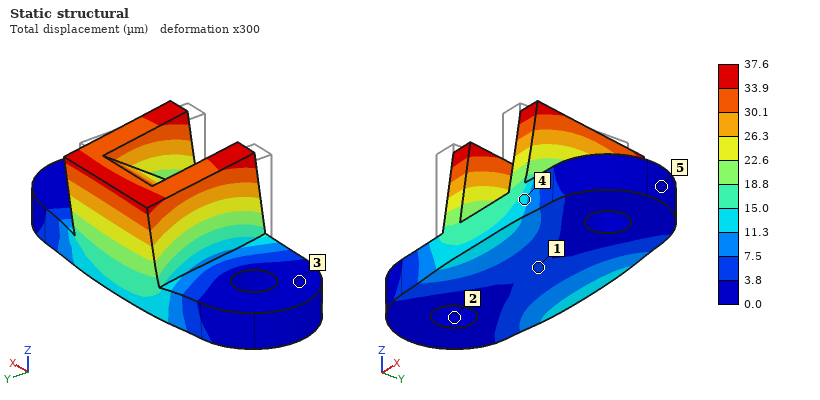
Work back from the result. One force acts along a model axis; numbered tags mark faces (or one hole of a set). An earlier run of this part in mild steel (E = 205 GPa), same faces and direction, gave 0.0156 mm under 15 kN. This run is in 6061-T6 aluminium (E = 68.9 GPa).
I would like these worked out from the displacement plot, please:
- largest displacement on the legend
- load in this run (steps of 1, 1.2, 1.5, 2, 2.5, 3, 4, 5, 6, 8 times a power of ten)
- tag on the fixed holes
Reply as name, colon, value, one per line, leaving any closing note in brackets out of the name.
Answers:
largest displacement on the legend: 37.6 µm
load in this run: 12 kN
tag on the fixed holes: 2
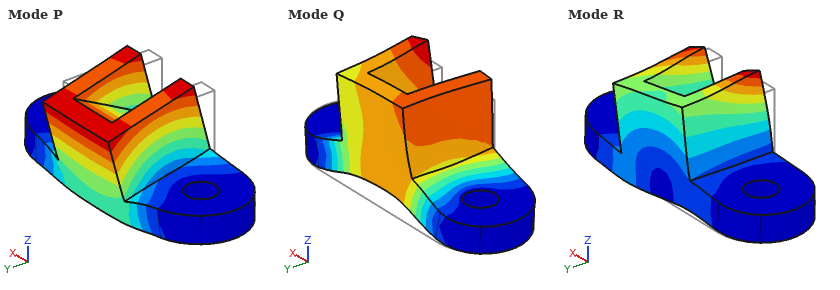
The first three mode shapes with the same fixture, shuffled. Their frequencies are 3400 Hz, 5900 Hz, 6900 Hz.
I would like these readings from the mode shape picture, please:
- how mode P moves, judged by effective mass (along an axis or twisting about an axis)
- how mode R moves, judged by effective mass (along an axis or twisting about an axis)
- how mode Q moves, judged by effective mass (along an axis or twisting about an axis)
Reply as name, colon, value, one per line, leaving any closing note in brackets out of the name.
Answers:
how mode P moves, judged by effective mass: along Y
how mode R moves, judged by effective mass: along X
how mode Q moves, judged by effective mass: along Z
